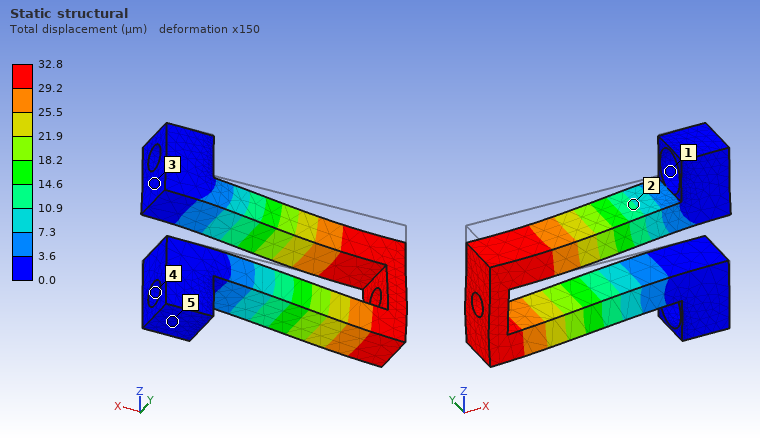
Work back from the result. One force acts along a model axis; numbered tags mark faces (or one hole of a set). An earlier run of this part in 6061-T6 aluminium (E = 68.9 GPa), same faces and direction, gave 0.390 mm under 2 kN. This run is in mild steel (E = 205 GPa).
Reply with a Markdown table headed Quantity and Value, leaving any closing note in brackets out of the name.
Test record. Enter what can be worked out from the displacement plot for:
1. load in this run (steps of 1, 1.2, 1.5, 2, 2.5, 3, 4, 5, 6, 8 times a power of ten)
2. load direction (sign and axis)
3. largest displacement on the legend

| Quantity | Value |
|---|---|
| load in this run | 500 N |
| load direction | -Z |
| largest displacement on the legend | 32.8 µm |
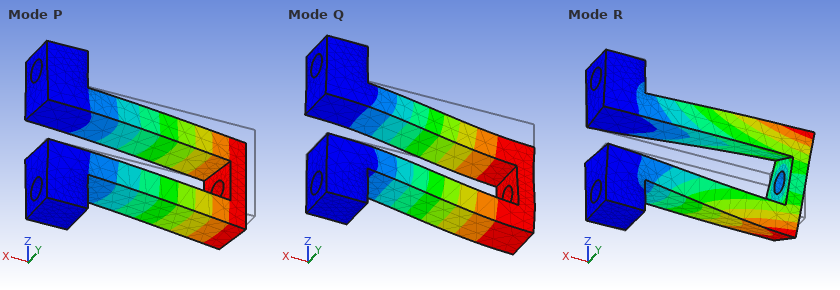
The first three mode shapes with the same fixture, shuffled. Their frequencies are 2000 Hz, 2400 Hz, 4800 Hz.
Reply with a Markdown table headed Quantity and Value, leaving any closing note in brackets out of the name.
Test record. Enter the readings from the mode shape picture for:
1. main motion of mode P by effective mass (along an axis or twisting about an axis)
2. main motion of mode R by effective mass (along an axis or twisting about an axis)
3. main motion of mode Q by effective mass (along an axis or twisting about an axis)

| Quantity | Value |
|---|---|
| main motion of mode P by effective mass | along Y |
| main motion of mode R by effective mass | twisting about X |
| main motion of mode Q by effective mass | along Z |
